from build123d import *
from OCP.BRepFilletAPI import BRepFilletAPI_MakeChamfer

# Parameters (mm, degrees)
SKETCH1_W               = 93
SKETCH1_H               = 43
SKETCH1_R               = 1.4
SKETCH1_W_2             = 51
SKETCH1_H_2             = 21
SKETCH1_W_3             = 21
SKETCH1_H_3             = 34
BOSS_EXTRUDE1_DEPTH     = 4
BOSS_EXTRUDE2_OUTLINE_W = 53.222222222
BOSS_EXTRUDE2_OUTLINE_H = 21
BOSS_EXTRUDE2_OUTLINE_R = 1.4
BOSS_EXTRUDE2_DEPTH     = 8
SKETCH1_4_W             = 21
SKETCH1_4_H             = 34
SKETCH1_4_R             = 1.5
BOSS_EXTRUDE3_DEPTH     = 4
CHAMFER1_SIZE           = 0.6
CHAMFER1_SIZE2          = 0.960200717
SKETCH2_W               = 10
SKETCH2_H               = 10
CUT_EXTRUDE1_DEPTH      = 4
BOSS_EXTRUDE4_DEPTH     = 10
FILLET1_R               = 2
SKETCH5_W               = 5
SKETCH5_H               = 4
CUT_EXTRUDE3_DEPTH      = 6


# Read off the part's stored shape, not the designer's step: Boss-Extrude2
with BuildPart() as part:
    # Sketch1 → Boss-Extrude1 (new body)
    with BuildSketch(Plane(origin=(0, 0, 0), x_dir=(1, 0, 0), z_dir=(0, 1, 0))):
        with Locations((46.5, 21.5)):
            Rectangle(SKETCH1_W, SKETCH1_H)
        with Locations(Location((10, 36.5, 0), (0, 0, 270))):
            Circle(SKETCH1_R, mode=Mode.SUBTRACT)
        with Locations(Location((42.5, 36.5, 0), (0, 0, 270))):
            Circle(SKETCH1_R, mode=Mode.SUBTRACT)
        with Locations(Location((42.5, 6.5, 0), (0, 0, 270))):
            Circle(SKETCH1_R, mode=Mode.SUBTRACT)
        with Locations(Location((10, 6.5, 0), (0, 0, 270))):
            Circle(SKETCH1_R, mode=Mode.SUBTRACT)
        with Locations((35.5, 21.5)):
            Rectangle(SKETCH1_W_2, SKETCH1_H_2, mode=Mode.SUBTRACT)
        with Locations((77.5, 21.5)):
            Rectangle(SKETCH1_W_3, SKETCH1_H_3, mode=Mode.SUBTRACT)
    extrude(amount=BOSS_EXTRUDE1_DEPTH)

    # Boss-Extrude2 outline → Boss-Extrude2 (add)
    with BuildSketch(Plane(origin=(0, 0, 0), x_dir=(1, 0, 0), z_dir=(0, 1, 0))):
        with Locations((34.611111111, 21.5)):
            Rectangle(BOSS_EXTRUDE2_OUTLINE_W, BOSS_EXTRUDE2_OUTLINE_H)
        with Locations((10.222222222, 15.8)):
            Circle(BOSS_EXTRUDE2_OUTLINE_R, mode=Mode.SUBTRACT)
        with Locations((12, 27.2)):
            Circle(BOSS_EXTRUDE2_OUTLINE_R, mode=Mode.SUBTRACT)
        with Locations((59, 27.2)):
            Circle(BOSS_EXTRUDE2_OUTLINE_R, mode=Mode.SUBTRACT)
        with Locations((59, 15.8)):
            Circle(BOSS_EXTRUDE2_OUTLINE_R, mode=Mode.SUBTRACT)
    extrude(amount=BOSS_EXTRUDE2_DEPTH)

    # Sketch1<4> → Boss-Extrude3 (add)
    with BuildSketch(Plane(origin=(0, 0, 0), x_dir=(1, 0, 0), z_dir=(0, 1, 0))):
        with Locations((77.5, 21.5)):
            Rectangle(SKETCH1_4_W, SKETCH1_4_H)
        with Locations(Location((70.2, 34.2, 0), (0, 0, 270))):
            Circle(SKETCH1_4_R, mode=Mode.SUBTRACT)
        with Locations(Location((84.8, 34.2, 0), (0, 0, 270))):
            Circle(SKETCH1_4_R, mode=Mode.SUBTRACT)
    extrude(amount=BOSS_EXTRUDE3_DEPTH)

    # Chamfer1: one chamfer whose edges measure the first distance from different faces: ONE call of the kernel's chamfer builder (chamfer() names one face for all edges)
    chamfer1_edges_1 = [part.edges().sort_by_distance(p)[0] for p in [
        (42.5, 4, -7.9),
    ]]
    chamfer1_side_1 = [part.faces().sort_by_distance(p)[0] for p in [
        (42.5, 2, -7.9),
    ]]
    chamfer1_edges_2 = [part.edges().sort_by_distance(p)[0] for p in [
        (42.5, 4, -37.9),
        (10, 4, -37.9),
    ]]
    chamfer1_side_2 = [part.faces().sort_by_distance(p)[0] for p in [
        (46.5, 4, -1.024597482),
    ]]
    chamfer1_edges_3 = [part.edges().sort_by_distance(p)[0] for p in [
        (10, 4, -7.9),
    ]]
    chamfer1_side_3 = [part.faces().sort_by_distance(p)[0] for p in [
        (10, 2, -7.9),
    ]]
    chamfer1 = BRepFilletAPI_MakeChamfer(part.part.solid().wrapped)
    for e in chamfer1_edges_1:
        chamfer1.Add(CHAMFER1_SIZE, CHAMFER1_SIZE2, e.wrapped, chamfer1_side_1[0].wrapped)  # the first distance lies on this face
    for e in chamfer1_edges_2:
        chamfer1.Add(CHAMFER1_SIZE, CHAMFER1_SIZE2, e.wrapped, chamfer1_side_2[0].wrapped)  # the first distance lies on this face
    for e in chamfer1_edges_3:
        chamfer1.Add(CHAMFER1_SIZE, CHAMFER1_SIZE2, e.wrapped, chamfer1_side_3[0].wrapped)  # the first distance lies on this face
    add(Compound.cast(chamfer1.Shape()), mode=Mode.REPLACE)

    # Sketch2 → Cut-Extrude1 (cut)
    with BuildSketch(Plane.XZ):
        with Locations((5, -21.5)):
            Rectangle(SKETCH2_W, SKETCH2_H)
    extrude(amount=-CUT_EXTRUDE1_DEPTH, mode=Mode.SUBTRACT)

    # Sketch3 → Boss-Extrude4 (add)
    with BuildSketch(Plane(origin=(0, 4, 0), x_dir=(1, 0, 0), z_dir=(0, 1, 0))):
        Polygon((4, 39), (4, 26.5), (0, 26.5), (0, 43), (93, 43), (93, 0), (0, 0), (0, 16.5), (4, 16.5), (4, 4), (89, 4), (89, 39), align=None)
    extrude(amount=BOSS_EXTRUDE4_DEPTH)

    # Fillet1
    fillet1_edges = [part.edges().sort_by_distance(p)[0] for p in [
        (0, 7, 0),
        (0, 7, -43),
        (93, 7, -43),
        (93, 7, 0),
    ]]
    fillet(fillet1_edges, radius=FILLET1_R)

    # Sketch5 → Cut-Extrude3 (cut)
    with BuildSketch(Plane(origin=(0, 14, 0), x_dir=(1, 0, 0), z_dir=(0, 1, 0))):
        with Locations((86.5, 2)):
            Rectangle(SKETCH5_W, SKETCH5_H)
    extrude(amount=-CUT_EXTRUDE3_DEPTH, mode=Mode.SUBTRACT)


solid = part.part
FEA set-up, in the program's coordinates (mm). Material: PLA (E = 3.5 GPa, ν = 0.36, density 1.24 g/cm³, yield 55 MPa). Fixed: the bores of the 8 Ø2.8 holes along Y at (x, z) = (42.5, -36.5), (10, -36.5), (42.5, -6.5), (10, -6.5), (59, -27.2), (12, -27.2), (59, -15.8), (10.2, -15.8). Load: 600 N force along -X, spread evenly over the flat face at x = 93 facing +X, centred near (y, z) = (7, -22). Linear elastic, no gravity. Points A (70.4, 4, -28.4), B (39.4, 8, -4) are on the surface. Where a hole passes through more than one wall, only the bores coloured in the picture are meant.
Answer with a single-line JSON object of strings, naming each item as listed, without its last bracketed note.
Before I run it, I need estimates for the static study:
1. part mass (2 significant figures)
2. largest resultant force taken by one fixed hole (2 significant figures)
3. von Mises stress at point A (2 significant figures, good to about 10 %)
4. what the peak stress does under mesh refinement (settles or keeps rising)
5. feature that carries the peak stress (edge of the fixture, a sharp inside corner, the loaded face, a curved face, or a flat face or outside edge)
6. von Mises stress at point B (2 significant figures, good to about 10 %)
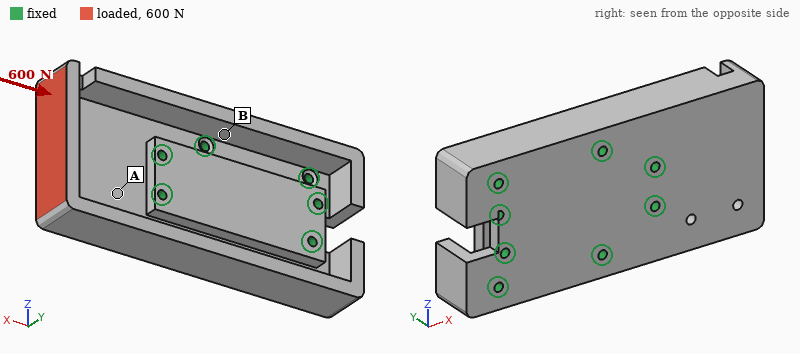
{"part mass": "36 g", "largest resultant force taken by one fixed hole": "150 N", "von Mises stress at point A": "5.3 MPa", "what the peak stress does under mesh refinement": "keeps rising", "feature that carries the peak stress": "a sharp inside corner", "von Mises stress at point B": "2.2 MPa"}
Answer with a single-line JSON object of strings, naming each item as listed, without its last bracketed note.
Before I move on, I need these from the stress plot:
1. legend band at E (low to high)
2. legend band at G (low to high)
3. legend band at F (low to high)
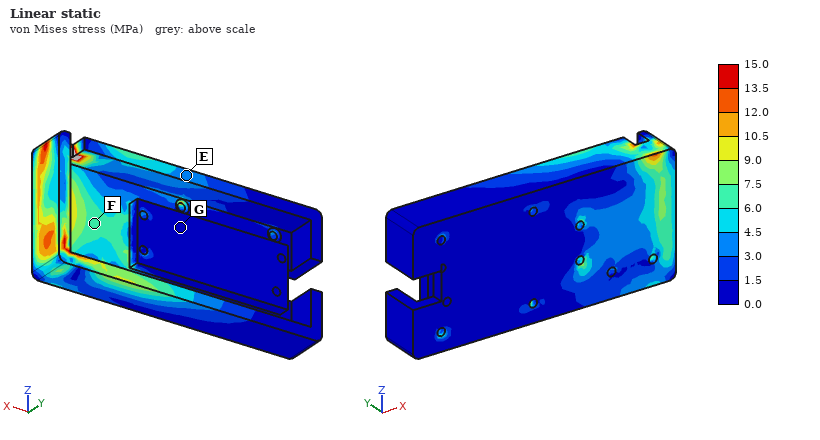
{"legend band at E": "3.0 to 4.5 MPa", "legend band at G": "0.0 to 1.5 MPa", "legend band at F": "6.0 to 7.5 MPa"}
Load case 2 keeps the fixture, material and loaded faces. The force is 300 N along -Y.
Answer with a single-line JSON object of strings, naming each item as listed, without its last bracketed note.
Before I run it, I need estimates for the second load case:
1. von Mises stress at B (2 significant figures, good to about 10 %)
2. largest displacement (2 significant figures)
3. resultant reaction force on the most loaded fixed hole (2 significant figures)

{"von Mises stress at B": "8.3 MPa", "largest displacement": "1.2 mm", "resultant reaction force on the most loaded fixed hole": "300 N"}
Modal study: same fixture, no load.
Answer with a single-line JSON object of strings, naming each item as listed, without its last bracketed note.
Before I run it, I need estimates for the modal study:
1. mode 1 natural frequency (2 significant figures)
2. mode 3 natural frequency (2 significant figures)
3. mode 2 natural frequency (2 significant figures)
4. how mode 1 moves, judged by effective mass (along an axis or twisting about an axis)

{"mode 1 natural frequency": "1200 Hz", "mode 3 natural frequency": "3400 Hz", "mode 2 natural frequency": "1500 Hz", "how mode 1 moves, judged by effective mass": "along Y"}
